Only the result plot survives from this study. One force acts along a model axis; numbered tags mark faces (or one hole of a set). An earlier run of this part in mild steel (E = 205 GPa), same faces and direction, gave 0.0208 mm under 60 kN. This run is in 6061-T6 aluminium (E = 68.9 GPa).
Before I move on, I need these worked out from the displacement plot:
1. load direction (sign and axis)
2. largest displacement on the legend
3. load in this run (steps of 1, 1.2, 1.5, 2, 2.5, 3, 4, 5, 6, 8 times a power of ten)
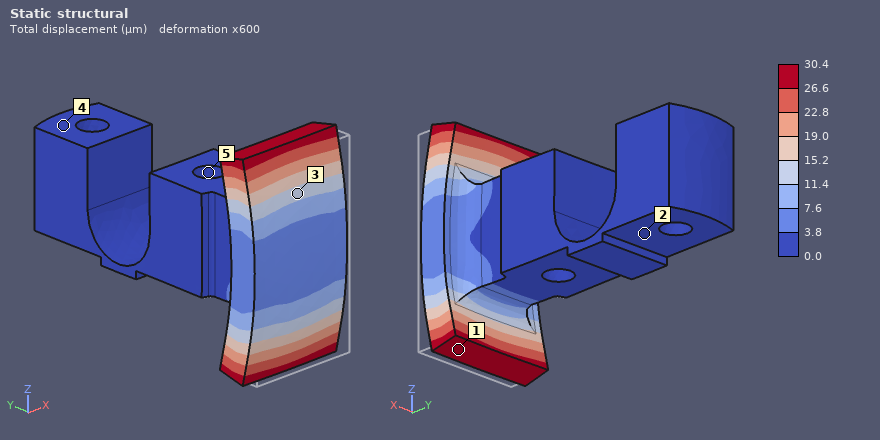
+Y
30.4 µm
30 kN
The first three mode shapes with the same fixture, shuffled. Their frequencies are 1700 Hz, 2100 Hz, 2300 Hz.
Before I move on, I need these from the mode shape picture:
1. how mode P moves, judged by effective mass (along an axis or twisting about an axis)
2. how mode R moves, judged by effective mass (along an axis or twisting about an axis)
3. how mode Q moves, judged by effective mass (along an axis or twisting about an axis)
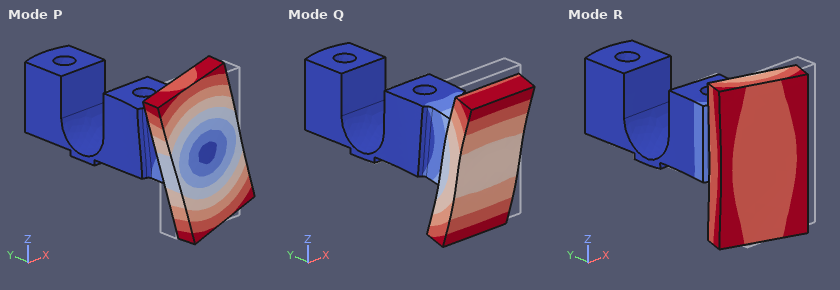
twisting about Y
along X
along Z
